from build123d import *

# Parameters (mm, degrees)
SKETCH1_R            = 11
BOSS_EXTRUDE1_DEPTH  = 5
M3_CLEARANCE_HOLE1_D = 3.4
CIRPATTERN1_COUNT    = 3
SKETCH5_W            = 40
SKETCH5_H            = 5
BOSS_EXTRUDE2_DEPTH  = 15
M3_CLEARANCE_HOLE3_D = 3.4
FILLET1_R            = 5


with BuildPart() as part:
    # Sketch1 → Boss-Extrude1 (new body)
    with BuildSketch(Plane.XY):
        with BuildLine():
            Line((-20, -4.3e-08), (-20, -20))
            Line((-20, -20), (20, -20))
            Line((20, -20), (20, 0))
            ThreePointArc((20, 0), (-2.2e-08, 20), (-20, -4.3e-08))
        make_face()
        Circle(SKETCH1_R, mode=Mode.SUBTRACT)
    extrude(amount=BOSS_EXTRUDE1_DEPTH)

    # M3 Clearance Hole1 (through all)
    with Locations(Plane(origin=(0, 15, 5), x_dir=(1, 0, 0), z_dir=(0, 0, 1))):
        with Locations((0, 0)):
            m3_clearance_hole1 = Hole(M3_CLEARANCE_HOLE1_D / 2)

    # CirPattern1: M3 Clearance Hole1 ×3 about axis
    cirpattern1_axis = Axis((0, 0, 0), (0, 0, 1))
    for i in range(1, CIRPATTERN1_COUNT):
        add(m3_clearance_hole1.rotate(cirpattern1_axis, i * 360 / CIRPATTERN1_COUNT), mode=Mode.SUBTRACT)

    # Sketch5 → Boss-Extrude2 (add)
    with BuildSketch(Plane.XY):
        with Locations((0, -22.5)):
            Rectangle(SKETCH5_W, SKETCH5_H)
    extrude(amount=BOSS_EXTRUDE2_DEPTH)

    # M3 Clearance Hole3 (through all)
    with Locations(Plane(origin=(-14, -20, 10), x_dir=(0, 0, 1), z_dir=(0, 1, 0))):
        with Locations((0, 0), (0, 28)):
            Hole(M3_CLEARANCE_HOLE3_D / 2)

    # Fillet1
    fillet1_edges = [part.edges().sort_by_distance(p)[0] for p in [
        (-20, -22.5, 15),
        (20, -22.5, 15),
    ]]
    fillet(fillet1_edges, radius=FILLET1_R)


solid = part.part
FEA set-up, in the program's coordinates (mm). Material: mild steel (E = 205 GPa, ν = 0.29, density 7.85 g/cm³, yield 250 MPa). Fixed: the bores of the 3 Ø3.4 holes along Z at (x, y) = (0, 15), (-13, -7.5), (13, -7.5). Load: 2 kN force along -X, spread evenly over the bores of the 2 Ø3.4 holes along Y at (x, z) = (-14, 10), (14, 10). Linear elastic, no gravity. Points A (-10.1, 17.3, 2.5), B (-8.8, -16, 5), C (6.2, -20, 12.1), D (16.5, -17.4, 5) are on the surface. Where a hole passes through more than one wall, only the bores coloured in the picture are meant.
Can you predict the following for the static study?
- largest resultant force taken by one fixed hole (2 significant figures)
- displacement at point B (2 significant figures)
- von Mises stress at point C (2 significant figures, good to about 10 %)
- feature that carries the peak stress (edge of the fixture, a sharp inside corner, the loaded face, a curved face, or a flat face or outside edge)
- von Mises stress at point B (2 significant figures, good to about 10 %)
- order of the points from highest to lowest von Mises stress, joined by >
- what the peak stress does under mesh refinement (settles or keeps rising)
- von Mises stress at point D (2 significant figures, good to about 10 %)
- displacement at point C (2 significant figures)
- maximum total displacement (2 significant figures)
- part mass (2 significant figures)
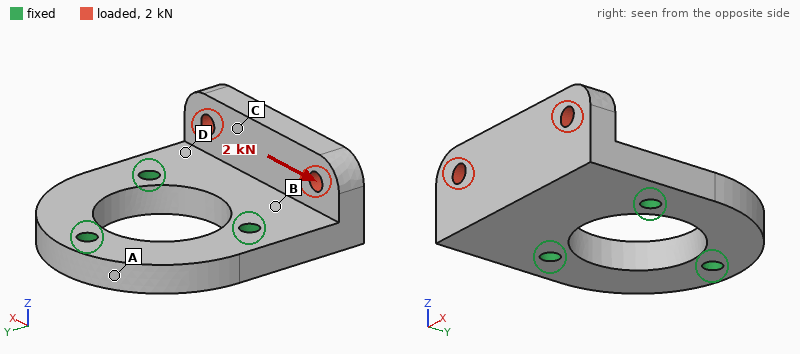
1.5 kN
4.0 µm
23 MPa
edge of the fixture
51 MPa
B > D > C > A
keeps rising
41 MPa
11 µm
17 µm
62 g
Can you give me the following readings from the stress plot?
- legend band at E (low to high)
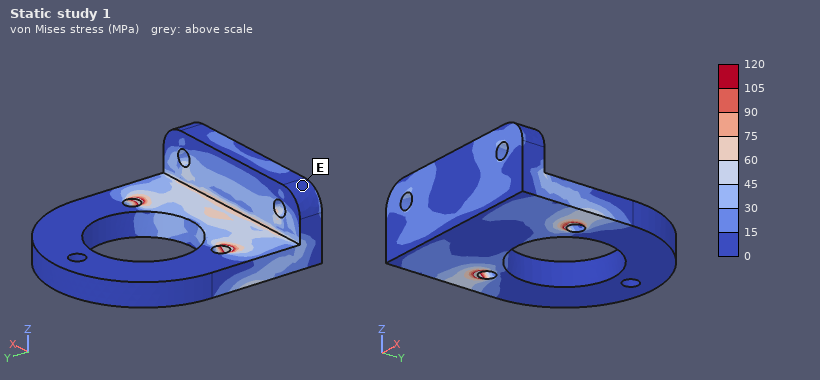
0 to 15 MPa
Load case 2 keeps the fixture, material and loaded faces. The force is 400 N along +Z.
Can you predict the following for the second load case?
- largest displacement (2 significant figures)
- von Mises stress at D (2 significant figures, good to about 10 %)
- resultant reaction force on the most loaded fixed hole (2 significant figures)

14 µm
15 MPa
210 N
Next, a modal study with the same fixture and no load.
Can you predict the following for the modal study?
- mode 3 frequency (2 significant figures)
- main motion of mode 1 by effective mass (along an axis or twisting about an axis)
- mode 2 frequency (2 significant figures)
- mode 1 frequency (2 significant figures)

19 kHz
along Z
11 kHz
6000 Hz
